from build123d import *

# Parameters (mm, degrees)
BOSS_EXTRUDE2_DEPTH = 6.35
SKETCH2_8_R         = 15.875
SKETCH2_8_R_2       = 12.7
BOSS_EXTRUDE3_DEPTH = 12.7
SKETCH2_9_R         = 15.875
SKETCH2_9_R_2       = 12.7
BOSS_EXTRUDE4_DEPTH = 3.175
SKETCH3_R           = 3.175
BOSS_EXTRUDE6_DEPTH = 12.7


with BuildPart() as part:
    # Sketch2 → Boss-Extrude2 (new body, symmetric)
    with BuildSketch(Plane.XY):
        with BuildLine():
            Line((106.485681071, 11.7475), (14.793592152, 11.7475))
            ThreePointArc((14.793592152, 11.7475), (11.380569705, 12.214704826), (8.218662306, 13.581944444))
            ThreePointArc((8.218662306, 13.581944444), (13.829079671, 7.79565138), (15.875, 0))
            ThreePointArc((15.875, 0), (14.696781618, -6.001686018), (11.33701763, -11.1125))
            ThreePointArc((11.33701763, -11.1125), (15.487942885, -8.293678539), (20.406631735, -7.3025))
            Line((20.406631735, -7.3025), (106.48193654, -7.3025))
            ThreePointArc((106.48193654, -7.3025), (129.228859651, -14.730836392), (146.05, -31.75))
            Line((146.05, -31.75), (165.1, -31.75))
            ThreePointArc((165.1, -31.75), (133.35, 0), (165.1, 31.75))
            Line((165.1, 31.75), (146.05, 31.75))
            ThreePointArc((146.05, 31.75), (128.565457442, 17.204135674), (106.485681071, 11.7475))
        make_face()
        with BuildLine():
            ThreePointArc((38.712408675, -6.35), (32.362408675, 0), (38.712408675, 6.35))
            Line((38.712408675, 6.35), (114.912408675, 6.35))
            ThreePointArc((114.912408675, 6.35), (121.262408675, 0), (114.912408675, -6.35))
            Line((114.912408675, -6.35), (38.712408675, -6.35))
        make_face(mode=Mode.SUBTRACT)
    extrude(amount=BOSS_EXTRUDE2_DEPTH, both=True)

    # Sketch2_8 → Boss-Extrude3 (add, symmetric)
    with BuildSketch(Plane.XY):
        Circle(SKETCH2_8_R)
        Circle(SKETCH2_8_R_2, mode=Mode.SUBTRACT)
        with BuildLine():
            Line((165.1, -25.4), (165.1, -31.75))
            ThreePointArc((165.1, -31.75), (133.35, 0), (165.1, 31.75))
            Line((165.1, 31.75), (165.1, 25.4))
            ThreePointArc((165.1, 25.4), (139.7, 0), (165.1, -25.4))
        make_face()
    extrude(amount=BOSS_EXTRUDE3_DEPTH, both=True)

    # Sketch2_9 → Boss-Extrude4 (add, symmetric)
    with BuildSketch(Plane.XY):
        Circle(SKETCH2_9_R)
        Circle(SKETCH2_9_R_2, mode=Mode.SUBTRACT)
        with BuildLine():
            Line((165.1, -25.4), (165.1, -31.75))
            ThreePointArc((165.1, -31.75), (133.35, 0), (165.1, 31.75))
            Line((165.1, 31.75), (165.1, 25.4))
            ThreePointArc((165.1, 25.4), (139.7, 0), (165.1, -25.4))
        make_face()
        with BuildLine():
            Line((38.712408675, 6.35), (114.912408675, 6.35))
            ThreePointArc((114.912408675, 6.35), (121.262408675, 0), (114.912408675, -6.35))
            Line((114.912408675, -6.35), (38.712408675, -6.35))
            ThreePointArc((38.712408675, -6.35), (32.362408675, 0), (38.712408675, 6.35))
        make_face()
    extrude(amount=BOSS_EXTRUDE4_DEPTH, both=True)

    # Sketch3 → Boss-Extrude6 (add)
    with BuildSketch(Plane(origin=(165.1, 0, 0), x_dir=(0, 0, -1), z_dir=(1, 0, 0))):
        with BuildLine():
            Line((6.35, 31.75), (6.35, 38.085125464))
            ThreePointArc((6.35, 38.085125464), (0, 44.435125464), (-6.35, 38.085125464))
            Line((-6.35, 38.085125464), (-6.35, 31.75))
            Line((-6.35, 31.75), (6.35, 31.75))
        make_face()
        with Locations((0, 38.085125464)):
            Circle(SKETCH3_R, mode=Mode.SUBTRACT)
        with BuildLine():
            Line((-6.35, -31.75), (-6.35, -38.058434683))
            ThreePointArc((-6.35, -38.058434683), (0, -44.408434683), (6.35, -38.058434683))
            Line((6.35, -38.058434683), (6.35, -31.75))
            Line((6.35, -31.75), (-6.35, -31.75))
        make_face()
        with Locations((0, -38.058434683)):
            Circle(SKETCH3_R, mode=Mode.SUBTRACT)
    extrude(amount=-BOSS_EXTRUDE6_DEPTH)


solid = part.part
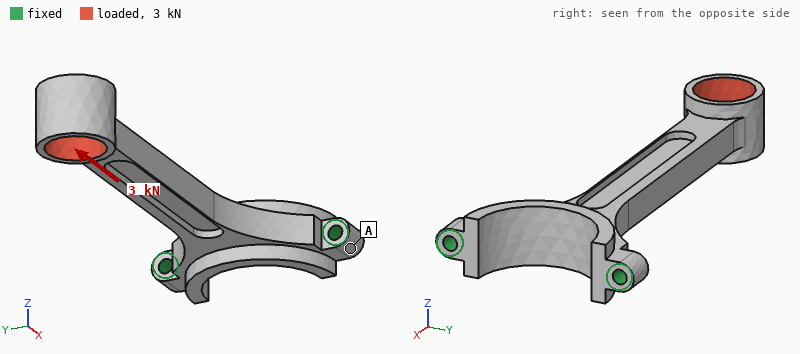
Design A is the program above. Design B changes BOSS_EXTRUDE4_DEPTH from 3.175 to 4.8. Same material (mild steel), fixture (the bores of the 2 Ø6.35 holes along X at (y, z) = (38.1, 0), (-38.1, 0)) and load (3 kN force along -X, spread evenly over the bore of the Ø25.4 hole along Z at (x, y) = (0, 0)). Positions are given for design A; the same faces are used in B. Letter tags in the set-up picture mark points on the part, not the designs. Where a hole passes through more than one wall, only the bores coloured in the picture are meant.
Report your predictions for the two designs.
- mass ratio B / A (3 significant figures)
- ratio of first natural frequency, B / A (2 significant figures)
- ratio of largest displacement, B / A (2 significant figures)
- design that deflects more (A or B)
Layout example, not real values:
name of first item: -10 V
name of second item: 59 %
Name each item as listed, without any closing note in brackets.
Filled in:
mass ratio B / A: 1.07
ratio of first natural frequency, B / A: 1.1
ratio of largest displacement, B / A: 0.77
design that deflects more: A
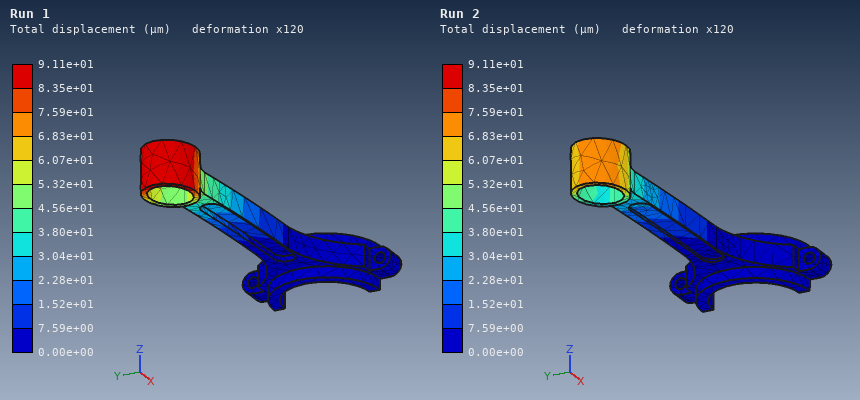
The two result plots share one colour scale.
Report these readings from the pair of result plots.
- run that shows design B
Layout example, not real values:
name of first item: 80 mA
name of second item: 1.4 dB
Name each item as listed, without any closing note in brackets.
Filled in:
run that shows design B: Run 2
